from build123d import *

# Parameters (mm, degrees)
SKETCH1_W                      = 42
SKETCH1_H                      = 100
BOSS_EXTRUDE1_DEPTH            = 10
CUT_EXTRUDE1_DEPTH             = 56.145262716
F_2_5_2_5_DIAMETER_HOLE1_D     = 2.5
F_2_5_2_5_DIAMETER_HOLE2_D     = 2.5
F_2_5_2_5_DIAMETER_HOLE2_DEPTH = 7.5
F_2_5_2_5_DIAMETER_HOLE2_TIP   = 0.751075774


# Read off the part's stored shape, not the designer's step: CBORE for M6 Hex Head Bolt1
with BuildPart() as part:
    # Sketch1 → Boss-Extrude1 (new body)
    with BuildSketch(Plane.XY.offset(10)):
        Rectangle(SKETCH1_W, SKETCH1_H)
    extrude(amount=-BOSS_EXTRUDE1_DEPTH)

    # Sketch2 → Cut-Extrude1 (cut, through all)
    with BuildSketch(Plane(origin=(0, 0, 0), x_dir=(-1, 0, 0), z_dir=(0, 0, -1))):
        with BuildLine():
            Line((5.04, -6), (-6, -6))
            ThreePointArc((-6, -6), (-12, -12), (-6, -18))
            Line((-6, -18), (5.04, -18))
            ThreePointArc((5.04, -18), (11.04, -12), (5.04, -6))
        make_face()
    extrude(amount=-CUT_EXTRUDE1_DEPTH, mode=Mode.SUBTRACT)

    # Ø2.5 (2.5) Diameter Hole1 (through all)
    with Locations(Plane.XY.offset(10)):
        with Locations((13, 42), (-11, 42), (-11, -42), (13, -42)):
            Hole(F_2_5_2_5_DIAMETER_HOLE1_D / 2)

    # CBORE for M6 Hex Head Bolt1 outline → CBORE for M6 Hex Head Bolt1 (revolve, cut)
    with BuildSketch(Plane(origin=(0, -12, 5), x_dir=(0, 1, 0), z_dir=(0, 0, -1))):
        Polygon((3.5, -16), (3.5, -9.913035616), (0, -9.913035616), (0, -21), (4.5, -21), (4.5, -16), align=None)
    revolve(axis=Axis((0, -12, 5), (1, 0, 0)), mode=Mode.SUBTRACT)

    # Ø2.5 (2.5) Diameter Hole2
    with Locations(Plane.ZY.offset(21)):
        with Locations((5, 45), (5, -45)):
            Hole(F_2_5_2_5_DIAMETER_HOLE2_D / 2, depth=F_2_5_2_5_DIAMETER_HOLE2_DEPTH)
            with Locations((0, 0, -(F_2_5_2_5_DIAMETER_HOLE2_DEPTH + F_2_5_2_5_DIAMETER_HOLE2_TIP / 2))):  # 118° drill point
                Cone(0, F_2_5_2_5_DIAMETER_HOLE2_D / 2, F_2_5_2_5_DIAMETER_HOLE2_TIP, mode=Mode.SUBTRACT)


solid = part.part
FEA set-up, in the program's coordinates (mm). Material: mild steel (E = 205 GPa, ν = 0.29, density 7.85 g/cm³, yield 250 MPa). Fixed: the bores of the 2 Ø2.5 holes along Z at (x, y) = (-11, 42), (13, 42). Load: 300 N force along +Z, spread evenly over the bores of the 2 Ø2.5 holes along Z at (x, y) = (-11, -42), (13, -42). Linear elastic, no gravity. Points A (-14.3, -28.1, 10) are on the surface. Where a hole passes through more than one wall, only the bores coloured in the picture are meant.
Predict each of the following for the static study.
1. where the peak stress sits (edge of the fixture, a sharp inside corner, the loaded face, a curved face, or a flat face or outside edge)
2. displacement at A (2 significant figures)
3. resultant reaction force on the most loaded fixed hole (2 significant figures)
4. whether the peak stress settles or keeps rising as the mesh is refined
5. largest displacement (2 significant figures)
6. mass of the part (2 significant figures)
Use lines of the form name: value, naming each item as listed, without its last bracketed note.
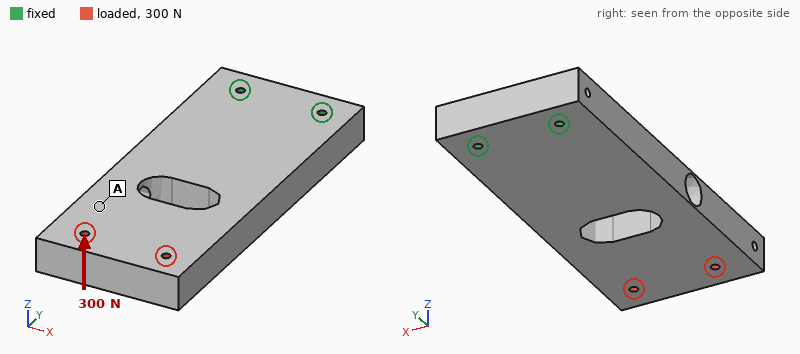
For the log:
where the peak stress sits: edge of the fixture
displacement at A: 0.082 mm
resultant reaction force on the most loaded fixed hole: 150 N
whether the peak stress settles or keeps rising as the mesh is refined: keeps rising
largest displacement: 0.13 mm
mass of the part: 300 g
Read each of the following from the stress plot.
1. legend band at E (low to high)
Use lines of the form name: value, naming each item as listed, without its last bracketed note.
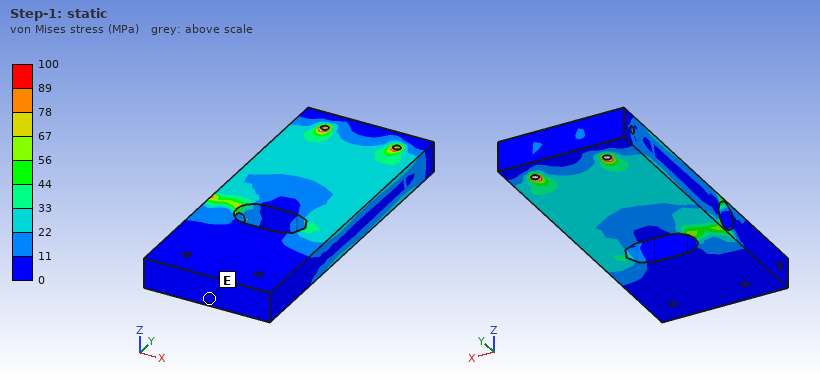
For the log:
legend band at E: 0 to 11 MPa
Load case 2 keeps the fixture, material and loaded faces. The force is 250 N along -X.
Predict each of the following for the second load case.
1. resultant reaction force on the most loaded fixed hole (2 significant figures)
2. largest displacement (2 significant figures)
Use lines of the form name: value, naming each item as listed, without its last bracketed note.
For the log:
resultant reaction force on the most loaded fixed hole: 850 N
largest displacement: 8.2 µm
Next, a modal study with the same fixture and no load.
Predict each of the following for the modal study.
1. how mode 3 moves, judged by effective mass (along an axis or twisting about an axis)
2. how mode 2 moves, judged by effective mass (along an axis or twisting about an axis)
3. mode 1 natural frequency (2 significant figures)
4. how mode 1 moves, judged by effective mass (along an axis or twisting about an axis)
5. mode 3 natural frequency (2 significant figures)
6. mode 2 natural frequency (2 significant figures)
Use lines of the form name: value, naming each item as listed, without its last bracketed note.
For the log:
how mode 3 moves, judged by effective mass: twisting about Y
how mode 2 moves, judged by effective mass: along X
mode 1 natural frequency: 890 Hz
how mode 1 moves, judged by effective mass: along Z
mode 3 natural frequency: 3700 Hz
mode 2 natural frequency: 3000 Hz
